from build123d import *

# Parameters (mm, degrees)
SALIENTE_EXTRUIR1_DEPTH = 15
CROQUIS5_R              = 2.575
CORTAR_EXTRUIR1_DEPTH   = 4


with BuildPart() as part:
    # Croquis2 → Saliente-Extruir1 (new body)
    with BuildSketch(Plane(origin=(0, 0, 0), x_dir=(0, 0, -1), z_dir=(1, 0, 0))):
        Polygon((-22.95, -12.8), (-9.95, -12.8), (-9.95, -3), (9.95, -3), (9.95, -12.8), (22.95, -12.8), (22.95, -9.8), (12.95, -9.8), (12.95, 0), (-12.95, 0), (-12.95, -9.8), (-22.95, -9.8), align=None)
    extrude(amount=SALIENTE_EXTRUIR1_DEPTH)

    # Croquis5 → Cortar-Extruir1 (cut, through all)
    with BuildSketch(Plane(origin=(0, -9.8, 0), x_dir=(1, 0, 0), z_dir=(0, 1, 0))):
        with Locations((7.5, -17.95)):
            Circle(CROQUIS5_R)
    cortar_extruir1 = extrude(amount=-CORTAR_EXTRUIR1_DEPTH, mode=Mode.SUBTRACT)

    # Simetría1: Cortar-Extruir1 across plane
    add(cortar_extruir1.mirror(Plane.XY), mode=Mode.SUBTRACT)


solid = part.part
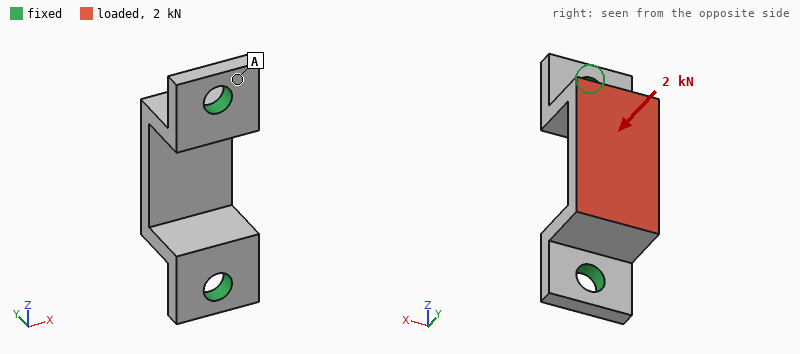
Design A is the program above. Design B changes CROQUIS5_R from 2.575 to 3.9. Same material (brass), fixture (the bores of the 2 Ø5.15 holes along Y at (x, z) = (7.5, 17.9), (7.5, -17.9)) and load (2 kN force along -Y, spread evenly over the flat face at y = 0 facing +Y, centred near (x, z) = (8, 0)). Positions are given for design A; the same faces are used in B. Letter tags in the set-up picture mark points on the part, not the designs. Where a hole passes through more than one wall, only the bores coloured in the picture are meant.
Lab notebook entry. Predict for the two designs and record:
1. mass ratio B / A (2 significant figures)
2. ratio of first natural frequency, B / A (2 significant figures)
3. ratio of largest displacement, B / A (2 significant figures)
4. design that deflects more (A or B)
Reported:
0.94
1.3
0.91
A
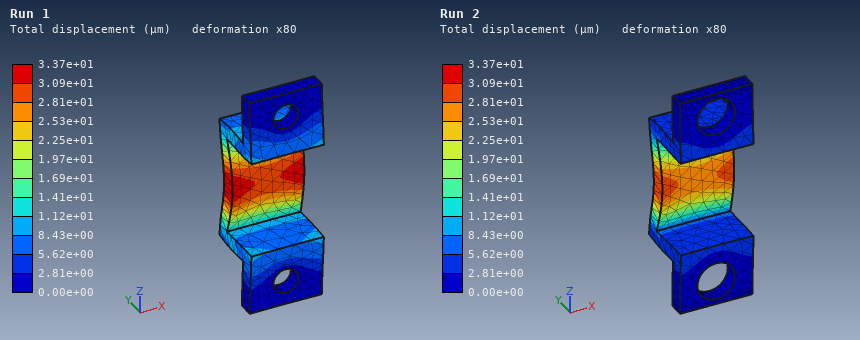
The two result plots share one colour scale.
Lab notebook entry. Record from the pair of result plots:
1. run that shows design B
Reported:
Run 2
